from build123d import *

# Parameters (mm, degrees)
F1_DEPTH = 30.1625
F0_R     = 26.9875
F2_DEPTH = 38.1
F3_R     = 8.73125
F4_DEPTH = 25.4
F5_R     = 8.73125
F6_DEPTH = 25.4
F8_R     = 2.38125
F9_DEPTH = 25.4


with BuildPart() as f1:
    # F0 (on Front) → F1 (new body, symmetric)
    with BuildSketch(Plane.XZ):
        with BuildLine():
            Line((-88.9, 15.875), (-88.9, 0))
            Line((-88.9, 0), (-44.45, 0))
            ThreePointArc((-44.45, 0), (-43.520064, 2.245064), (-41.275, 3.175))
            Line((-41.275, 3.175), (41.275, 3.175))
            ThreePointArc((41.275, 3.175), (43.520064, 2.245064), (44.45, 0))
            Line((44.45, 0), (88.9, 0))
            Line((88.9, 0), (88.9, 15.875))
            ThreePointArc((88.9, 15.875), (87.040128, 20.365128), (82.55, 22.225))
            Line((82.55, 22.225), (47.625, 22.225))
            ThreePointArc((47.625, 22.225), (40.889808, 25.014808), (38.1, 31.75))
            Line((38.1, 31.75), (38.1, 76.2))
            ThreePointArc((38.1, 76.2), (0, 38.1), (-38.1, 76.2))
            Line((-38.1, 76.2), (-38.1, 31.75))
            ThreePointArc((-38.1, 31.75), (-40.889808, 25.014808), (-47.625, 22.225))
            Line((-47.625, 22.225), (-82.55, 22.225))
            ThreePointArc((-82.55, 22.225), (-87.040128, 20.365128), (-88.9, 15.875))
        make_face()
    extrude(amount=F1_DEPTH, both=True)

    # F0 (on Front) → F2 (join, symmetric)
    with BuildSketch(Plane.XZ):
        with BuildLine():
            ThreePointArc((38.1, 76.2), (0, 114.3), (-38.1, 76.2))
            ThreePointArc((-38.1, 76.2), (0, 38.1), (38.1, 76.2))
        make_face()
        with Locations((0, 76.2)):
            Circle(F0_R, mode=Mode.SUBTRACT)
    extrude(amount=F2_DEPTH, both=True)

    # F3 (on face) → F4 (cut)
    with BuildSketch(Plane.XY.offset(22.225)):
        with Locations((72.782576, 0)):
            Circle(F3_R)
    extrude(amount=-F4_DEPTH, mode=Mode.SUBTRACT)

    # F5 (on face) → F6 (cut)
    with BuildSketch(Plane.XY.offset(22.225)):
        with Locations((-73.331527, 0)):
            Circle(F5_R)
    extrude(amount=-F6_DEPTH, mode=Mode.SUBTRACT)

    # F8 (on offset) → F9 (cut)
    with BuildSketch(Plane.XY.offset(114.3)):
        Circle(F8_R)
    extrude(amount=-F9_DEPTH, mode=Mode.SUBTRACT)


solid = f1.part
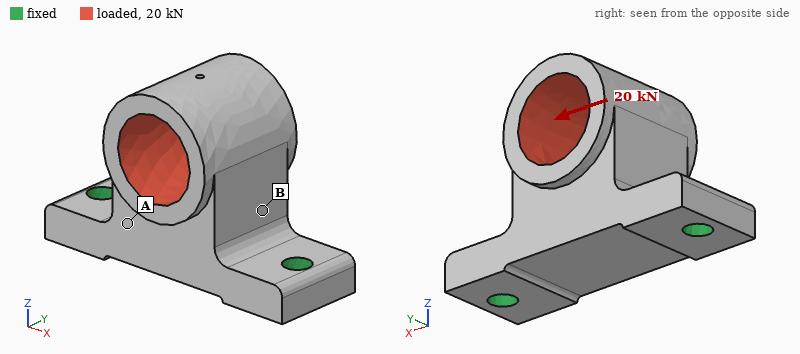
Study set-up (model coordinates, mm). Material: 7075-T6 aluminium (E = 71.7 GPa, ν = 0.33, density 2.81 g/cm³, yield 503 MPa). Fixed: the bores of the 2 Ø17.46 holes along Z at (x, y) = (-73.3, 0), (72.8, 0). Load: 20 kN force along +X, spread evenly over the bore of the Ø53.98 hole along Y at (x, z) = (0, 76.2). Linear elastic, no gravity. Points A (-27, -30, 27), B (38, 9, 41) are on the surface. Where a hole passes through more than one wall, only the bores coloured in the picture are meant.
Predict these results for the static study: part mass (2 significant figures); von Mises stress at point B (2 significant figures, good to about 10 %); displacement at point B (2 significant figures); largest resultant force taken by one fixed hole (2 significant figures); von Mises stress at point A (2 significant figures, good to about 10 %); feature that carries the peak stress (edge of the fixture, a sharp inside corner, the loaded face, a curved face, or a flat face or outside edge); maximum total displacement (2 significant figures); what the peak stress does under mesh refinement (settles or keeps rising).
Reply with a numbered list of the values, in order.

1. 1.4 kg
2. 28 MPa
3. 0.036 mm
4. 15 kN
5. 13 MPa
6. edge of the fixture
7. 0.15 mm
8. keeps rising
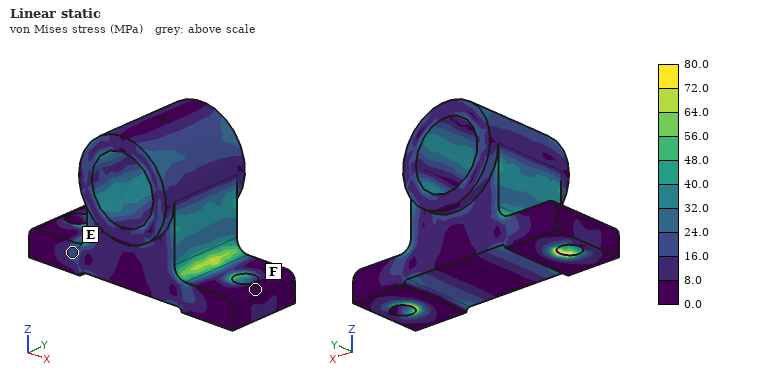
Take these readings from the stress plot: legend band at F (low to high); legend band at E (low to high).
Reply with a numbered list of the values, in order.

1. 0.0 to 8.0 MPa
2. 16.0 to 24.0 MPa
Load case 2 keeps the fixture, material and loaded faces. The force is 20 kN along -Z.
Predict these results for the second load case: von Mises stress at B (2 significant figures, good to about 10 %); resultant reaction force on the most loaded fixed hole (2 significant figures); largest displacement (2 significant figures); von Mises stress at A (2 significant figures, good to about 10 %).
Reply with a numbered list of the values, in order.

1. 13 MPa
2. 11 kN
3. 45 µm
4. 9.1 MPa
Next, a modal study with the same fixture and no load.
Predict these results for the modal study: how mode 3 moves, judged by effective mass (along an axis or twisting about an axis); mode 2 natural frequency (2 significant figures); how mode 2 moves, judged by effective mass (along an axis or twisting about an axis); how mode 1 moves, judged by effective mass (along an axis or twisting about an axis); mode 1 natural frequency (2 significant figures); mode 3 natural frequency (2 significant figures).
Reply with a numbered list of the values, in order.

1. along Z
2. 2900 Hz
3. along X
4. along Y
5. 1400 Hz
6. 3800 Hz
